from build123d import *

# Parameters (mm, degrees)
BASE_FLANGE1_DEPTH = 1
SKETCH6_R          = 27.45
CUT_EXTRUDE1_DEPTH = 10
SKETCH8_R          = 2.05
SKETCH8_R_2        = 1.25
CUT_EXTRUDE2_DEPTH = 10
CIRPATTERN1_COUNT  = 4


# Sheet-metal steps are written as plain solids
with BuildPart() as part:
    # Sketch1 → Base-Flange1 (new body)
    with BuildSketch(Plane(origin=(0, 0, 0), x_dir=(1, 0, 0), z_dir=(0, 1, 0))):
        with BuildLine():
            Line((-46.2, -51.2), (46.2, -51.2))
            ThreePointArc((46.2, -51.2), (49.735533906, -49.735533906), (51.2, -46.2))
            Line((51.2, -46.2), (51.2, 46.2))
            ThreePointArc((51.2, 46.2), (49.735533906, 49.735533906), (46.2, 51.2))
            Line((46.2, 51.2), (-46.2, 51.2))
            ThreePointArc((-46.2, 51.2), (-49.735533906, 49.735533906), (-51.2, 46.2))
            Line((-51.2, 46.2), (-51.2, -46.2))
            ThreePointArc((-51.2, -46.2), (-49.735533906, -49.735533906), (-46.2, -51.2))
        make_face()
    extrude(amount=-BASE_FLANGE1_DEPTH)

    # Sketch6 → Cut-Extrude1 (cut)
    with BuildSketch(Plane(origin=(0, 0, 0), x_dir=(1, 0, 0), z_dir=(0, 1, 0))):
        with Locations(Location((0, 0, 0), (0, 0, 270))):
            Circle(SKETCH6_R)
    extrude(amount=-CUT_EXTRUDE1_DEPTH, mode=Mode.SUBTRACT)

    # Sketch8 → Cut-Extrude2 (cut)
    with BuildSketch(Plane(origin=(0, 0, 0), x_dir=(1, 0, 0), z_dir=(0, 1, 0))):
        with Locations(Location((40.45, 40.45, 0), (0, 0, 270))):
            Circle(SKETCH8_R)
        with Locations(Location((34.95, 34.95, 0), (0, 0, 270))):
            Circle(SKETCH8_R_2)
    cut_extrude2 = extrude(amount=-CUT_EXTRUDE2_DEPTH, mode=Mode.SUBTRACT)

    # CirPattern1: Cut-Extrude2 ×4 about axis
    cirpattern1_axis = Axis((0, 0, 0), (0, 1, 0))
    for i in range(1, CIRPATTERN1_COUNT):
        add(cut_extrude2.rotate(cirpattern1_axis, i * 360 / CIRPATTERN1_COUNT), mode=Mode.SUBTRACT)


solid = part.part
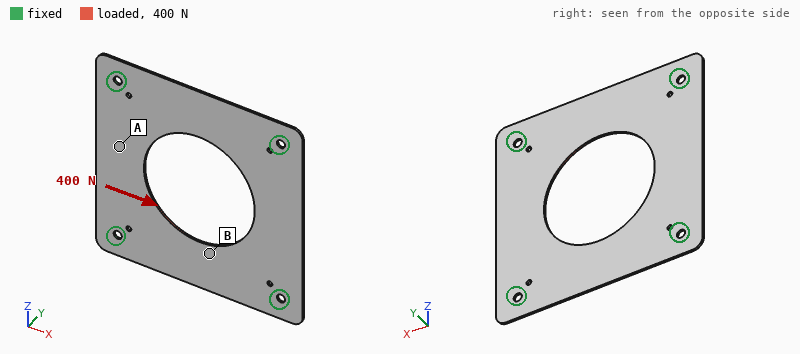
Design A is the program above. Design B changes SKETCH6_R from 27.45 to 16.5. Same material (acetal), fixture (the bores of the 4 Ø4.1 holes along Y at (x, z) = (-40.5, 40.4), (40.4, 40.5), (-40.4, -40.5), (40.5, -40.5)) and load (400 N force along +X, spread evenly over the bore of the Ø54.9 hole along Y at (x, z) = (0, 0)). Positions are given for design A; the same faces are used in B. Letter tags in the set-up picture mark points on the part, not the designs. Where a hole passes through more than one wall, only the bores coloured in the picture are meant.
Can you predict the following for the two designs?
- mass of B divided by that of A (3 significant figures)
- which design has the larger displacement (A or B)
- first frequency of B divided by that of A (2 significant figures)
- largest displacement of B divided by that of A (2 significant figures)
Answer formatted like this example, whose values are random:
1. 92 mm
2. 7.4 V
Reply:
1. 1.19
2. A
3. 0.79
4. 0.90
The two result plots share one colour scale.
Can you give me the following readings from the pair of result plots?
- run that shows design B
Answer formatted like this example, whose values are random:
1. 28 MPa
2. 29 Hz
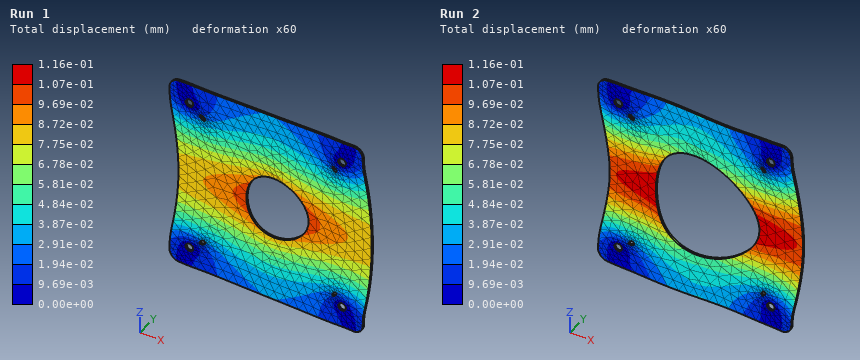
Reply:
1. Run 1
